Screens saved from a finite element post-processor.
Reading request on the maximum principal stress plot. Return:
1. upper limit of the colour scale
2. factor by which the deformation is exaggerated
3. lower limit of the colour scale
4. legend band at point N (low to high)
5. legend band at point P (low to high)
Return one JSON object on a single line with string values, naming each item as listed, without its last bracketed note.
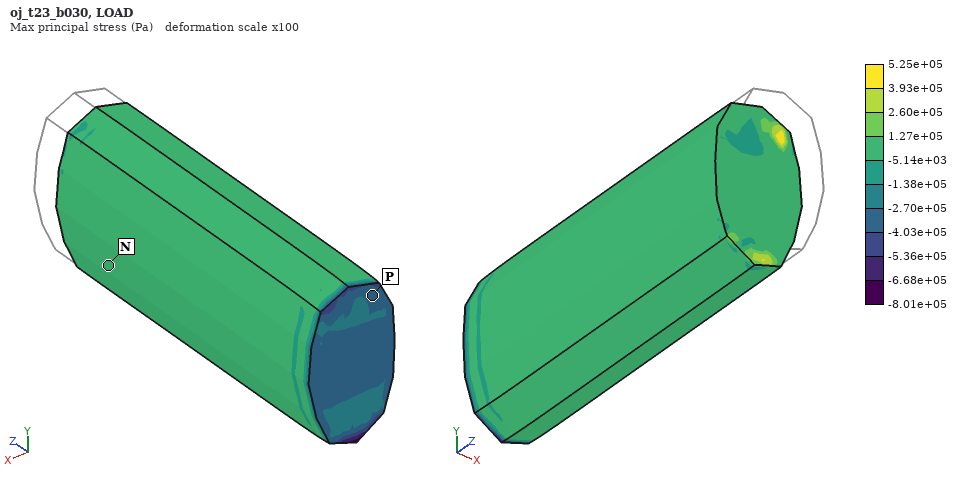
{"upper limit of the colour scale": "5.25e+05 Pa", "factor by which the deformation is exaggerated": "100", "lower limit of the colour scale": "-8.01e+05 Pa", "legend band at point N": "-5.14e+03 to 1.27e+05 Pa", "legend band at point P": "-4.03e+05 to -2.70e+05 Pa"}
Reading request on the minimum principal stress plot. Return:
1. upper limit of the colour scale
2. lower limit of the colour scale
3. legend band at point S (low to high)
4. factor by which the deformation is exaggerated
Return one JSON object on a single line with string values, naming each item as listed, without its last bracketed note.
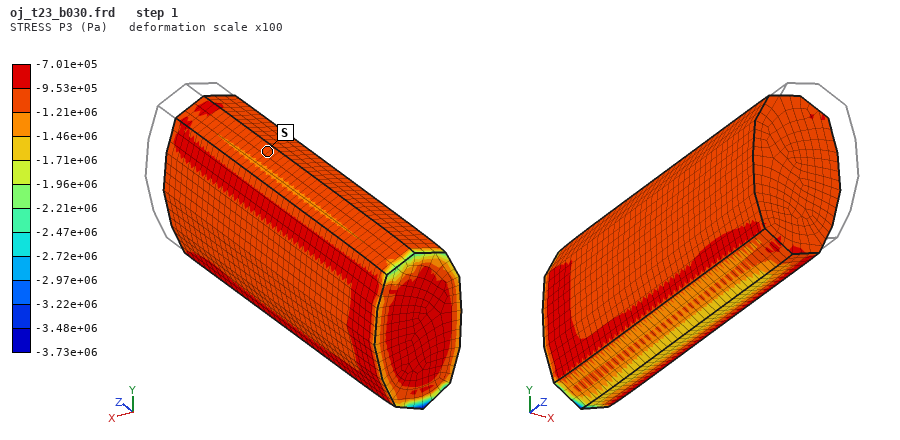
{"upper limit of the colour scale": "-7.01e+05 Pa", "lower limit of the colour scale": "-3.73e+06 Pa", "legend band at point S": "-1.21e+06 to -9.53e+05 Pa", "factor by which the deformation is exaggerated": "100"}
